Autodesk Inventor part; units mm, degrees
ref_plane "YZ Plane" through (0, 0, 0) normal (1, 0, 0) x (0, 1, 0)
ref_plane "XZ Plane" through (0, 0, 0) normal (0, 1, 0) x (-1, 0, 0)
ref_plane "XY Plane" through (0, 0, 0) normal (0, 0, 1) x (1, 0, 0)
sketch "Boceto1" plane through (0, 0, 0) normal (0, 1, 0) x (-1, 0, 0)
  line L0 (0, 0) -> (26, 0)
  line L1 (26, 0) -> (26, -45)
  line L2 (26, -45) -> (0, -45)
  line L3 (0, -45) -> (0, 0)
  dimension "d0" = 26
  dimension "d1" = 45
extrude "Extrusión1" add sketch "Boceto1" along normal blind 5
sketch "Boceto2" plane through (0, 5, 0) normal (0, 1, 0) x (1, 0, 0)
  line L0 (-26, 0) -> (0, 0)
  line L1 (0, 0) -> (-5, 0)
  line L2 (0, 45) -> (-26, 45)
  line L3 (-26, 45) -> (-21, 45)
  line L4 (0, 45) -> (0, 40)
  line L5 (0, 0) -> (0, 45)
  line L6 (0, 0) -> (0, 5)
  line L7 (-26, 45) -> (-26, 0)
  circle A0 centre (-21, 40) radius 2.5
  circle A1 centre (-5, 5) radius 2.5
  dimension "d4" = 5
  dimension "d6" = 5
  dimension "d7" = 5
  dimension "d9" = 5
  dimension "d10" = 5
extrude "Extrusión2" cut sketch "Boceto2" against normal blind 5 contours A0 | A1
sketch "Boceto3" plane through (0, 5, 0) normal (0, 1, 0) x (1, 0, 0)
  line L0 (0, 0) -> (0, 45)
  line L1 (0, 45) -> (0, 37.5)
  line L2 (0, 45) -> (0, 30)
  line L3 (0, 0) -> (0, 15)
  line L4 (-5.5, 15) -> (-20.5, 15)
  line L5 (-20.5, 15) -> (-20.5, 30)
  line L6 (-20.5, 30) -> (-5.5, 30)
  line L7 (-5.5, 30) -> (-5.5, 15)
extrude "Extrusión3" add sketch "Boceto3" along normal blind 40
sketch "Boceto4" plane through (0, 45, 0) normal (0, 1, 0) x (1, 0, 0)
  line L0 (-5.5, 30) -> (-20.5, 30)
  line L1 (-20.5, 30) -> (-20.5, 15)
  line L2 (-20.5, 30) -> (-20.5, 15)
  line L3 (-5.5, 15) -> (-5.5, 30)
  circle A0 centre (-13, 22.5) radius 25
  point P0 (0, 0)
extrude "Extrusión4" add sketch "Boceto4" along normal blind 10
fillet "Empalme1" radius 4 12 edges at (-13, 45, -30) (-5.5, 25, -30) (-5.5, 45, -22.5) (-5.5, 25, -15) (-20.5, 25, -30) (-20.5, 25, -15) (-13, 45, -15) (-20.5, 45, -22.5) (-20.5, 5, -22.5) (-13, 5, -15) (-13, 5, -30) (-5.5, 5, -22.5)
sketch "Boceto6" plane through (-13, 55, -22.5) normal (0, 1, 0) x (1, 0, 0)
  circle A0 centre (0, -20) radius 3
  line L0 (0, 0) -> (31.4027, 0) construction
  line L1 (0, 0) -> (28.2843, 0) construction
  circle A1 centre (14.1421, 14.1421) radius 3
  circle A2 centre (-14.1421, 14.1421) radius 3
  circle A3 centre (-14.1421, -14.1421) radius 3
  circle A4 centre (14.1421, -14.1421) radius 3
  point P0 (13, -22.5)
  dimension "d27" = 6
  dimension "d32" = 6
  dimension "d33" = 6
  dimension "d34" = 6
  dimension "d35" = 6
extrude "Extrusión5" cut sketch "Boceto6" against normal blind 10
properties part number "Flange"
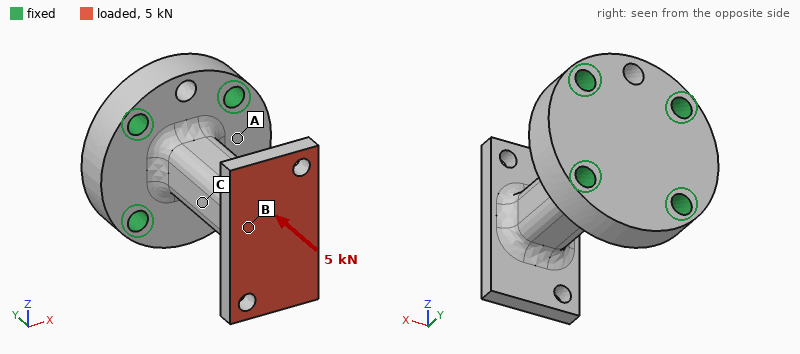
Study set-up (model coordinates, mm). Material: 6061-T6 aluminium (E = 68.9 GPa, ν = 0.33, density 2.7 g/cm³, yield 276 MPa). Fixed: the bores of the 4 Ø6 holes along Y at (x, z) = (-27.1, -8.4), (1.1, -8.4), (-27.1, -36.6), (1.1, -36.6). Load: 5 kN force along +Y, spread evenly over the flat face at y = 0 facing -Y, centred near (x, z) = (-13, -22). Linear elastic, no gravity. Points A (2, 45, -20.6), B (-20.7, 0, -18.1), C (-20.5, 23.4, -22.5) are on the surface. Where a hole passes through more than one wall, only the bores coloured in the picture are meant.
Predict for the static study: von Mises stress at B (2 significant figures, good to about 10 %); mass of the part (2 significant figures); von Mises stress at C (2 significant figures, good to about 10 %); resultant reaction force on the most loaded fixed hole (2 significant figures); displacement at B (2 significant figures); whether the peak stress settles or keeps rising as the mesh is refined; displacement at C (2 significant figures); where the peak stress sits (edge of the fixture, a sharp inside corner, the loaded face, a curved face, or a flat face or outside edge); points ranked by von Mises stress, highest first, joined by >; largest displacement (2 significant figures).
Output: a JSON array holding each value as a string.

["60 MPa", "88 g", "24 MPa", "1.3 kN", "20 µm", "keeps rising", "13 µm", "a sharp inside corner", "B > C > A", "84 µm"]
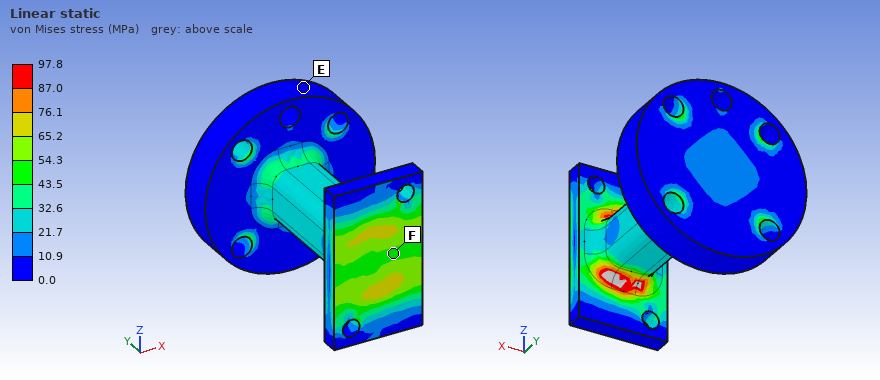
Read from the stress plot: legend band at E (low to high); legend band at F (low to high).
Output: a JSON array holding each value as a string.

["0.0 to 10.9 MPa", "43.5 to 54.3 MPa"]
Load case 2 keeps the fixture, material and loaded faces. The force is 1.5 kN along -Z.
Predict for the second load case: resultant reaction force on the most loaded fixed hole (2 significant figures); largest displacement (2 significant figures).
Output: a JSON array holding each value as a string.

["1.5 kN", "0.28 mm"]
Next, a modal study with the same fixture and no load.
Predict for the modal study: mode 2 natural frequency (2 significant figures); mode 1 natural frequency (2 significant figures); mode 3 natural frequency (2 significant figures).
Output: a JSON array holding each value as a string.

["3000 Hz", "2900 Hz", "5400 Hz"]
